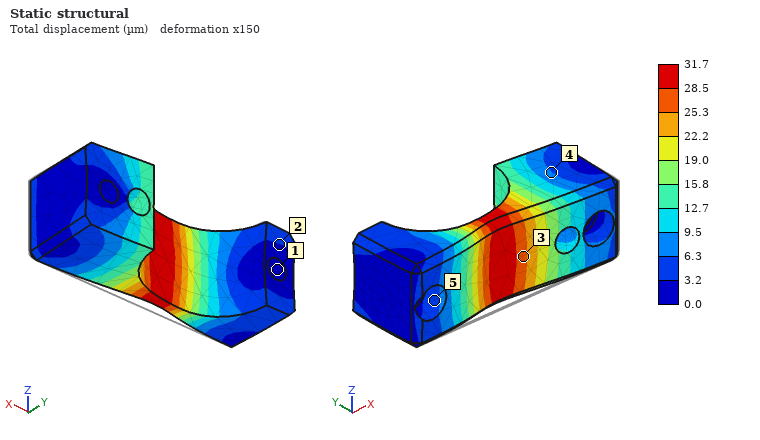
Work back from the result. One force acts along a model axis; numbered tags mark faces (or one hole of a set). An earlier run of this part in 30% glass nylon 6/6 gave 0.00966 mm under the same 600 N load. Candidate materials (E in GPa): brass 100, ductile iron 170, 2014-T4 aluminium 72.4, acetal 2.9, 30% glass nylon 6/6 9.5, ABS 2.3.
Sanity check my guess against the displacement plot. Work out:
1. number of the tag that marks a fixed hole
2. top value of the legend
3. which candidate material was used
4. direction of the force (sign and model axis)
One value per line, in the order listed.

1
31.7 µm
acetal
+Y
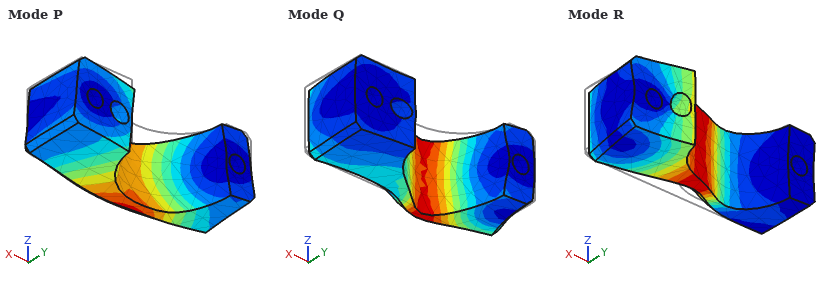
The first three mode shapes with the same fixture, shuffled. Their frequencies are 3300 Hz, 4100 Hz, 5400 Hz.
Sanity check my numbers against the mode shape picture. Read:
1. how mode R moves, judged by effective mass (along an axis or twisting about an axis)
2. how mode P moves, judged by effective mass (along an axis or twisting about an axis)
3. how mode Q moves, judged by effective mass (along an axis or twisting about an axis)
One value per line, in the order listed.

along Y
along Z
along X
